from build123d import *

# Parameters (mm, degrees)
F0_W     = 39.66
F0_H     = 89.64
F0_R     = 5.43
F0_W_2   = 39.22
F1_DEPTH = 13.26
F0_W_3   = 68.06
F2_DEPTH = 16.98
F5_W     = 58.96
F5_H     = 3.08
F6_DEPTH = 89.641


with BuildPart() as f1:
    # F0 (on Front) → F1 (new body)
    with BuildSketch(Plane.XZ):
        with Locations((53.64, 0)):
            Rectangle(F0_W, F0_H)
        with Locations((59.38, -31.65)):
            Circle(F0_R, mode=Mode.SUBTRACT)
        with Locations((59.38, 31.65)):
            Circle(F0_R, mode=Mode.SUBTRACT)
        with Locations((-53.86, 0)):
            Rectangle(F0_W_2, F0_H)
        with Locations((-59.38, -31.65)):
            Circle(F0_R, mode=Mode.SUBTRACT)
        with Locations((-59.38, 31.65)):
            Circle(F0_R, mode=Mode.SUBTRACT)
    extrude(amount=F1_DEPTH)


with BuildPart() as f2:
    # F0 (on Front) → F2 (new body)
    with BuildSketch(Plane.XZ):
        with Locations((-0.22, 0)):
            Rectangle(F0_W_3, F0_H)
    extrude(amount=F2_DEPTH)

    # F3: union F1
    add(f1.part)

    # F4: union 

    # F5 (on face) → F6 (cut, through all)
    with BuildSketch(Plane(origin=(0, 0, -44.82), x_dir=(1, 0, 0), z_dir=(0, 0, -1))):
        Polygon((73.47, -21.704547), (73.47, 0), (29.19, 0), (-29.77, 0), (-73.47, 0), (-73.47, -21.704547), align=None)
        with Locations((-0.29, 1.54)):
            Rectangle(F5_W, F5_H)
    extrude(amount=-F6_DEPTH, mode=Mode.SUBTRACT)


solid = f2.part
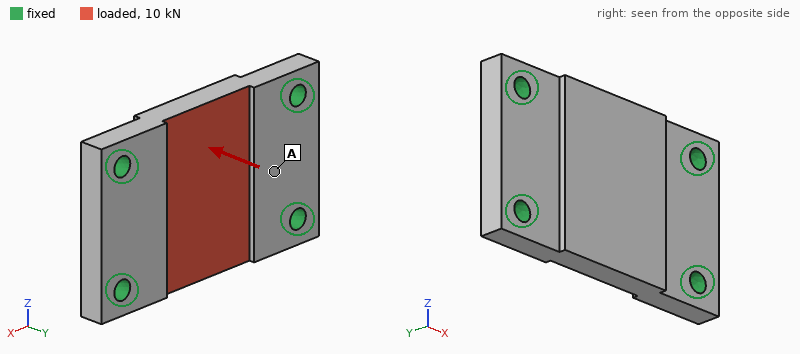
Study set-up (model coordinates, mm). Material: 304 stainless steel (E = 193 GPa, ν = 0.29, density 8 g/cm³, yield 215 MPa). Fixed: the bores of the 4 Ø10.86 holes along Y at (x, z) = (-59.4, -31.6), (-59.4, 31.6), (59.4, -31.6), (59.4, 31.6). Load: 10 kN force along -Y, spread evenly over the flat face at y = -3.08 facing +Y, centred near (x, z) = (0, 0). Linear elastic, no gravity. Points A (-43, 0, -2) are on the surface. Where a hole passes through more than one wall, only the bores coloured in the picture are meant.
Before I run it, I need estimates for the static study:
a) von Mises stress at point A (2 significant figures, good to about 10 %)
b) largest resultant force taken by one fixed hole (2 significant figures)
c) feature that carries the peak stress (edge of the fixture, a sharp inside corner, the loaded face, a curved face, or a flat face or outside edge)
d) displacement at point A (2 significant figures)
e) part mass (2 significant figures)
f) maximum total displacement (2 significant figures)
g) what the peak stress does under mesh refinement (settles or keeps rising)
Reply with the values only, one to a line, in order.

10 MPa
3.6 kN
edge of the fixture
7.6 µm
1.4 kg
21 µm
keeps rising
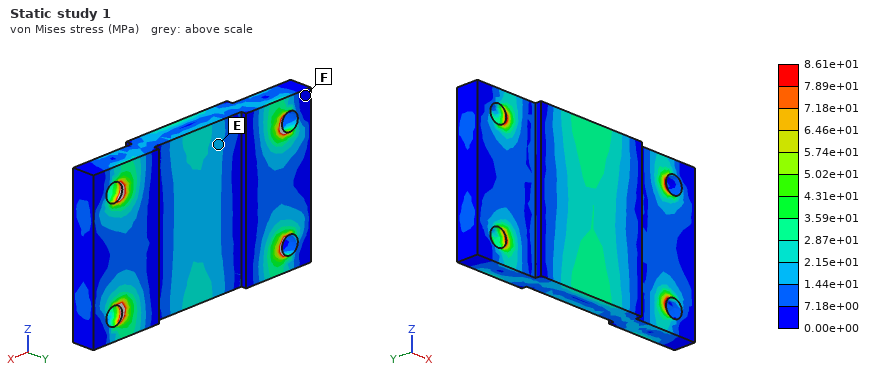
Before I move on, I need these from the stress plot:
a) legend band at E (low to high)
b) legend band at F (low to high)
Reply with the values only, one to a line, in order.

1.44e+01 to 2.15e+01 MPa
0.00e+00 to 7.18e+00 MPa
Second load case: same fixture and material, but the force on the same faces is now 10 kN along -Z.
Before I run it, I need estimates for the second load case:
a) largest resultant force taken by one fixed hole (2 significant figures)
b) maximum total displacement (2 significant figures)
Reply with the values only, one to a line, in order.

3.0 kN
5.9 µm
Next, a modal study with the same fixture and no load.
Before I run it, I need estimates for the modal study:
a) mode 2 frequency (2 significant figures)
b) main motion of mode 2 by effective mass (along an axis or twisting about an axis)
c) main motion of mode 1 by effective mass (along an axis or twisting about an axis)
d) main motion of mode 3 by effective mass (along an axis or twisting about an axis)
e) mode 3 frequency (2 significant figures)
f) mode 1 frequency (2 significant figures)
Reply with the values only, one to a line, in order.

6200 Hz
twisting about X
along Y
twisting about Z
10 kHz
4500 Hz
